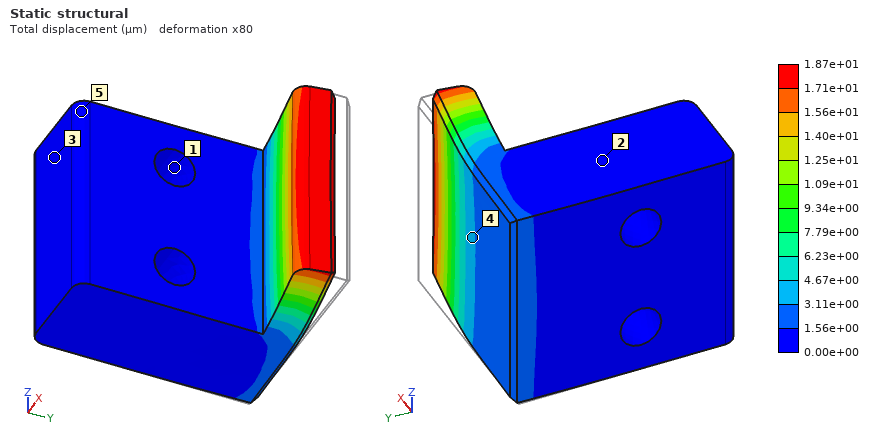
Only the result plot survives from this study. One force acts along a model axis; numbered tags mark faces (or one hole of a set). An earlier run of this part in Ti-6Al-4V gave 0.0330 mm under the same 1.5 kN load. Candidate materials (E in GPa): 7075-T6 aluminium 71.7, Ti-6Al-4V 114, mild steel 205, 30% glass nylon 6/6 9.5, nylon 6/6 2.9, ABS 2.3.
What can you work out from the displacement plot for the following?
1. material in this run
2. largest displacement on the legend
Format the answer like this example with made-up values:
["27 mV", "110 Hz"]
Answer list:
["mild steel", "1.87e+01 µm"]
